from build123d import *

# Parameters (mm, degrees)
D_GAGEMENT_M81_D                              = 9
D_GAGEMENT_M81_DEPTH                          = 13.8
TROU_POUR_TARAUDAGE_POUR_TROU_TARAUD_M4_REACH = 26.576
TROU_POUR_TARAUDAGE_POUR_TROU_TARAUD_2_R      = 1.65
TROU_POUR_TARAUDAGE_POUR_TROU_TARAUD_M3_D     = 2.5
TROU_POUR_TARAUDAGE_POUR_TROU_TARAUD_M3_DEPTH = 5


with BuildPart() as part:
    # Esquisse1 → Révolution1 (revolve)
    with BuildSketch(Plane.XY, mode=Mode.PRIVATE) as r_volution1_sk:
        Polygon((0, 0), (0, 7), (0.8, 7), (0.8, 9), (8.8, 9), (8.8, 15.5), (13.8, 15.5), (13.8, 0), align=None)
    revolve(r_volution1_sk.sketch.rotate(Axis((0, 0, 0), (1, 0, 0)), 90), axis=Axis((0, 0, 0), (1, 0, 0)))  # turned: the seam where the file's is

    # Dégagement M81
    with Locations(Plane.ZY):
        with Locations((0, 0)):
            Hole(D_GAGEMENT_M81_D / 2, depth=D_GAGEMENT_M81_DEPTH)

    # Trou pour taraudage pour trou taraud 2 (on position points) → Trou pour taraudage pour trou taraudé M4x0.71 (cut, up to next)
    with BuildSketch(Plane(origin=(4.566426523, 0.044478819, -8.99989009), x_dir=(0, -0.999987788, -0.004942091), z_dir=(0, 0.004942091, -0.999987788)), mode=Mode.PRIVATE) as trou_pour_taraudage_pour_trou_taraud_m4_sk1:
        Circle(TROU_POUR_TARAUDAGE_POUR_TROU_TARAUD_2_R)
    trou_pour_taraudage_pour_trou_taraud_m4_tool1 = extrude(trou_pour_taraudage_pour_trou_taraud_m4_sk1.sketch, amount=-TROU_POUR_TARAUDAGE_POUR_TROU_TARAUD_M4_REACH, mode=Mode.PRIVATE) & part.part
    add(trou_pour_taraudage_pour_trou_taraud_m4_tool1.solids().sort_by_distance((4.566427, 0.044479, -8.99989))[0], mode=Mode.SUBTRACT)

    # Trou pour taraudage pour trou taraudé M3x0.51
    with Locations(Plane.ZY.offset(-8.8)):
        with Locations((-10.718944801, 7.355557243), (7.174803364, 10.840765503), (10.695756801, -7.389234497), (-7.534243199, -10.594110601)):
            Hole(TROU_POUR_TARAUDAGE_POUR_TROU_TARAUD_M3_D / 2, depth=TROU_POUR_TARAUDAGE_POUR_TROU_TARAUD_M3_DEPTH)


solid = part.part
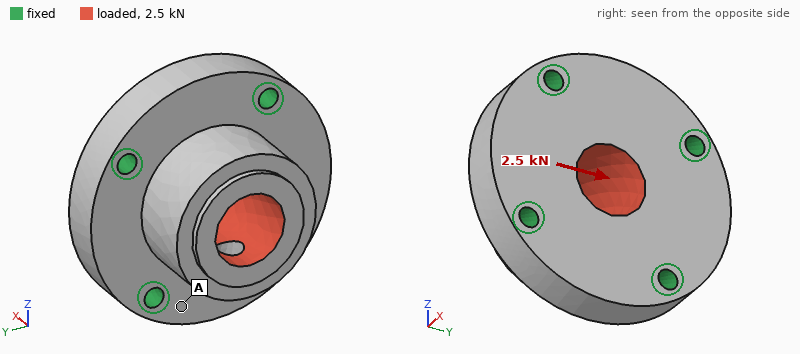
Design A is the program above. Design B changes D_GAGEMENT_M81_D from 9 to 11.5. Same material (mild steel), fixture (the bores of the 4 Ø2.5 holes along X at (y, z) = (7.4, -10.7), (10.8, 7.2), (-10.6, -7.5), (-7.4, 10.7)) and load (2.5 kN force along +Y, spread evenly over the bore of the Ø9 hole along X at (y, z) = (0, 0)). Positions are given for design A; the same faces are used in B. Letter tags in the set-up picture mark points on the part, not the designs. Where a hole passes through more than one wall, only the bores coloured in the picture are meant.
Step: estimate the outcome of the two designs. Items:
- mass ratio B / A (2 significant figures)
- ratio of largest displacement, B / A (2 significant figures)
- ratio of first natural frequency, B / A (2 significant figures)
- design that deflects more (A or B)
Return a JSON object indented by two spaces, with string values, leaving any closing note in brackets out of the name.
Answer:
{
  "mass ratio B / A": "0.89",
  "ratio of largest displacement, B / A": "1.2",
  "ratio of first natural frequency, B / A": "1.0",
  "design that deflects more": "B"
}
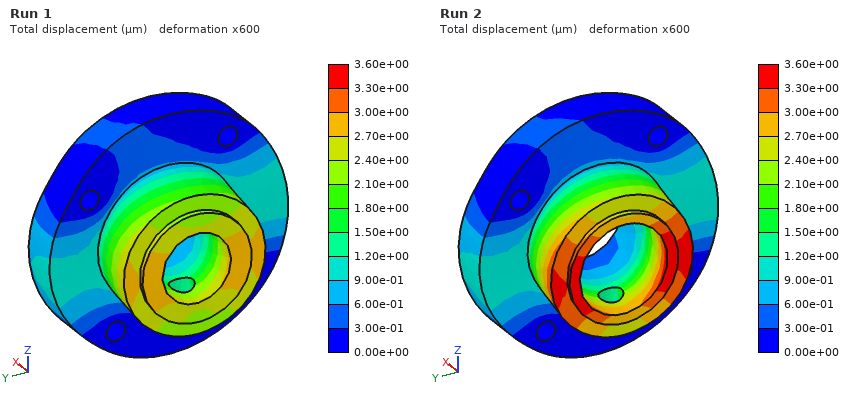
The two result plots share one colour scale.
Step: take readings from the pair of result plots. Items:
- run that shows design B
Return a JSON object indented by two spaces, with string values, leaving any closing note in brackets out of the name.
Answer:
{
  "run that shows design B": "Run 2"
}
